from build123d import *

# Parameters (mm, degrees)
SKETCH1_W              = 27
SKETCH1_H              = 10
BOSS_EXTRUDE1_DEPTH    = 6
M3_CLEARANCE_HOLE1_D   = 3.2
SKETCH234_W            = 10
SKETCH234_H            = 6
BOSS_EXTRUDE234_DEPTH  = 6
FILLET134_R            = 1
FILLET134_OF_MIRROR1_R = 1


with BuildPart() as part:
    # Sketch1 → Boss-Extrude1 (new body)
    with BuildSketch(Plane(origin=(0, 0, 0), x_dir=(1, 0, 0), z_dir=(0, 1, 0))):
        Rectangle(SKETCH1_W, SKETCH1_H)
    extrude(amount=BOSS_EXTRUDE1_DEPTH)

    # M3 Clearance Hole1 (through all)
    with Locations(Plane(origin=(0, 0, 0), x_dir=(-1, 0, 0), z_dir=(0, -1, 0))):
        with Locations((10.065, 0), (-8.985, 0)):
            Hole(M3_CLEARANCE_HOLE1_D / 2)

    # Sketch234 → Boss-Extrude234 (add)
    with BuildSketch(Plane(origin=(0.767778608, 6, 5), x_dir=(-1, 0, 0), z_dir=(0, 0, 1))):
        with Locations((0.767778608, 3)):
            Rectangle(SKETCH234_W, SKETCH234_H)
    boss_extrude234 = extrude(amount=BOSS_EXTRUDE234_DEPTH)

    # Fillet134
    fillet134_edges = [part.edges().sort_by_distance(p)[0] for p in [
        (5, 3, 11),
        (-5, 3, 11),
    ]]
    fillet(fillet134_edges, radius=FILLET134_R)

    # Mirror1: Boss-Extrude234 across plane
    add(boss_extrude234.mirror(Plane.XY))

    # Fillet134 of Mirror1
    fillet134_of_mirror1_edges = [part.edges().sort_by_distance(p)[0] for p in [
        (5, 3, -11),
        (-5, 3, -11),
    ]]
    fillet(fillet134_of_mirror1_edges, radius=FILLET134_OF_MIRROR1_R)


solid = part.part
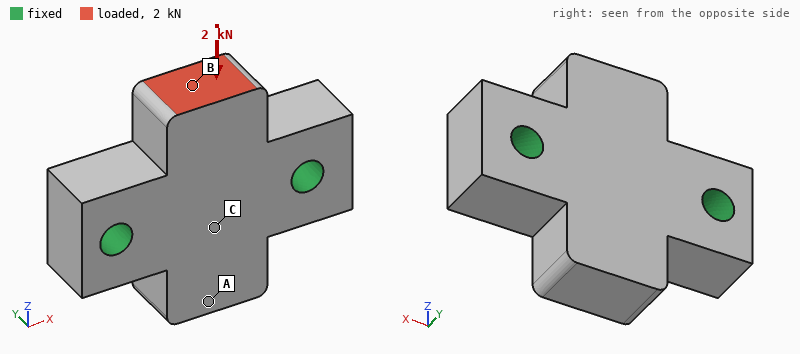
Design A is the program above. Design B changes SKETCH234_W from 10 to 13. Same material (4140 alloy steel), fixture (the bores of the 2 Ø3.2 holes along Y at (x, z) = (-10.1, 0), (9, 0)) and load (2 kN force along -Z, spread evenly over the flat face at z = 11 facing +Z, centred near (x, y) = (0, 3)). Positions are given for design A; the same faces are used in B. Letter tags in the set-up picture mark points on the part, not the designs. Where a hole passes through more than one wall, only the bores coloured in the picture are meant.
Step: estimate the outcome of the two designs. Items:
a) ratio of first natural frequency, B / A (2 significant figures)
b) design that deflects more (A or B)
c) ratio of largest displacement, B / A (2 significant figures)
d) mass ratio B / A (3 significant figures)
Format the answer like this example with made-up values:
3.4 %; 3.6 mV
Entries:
1.00; A; 0.74; 1.10
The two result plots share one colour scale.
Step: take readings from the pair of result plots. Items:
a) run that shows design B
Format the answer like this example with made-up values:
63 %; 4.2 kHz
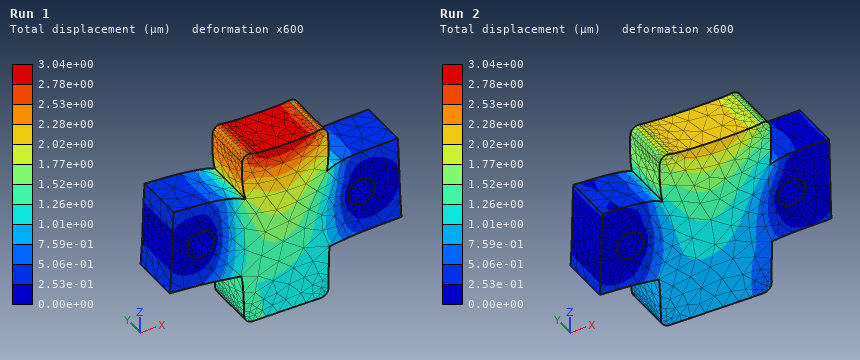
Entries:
Run 2
